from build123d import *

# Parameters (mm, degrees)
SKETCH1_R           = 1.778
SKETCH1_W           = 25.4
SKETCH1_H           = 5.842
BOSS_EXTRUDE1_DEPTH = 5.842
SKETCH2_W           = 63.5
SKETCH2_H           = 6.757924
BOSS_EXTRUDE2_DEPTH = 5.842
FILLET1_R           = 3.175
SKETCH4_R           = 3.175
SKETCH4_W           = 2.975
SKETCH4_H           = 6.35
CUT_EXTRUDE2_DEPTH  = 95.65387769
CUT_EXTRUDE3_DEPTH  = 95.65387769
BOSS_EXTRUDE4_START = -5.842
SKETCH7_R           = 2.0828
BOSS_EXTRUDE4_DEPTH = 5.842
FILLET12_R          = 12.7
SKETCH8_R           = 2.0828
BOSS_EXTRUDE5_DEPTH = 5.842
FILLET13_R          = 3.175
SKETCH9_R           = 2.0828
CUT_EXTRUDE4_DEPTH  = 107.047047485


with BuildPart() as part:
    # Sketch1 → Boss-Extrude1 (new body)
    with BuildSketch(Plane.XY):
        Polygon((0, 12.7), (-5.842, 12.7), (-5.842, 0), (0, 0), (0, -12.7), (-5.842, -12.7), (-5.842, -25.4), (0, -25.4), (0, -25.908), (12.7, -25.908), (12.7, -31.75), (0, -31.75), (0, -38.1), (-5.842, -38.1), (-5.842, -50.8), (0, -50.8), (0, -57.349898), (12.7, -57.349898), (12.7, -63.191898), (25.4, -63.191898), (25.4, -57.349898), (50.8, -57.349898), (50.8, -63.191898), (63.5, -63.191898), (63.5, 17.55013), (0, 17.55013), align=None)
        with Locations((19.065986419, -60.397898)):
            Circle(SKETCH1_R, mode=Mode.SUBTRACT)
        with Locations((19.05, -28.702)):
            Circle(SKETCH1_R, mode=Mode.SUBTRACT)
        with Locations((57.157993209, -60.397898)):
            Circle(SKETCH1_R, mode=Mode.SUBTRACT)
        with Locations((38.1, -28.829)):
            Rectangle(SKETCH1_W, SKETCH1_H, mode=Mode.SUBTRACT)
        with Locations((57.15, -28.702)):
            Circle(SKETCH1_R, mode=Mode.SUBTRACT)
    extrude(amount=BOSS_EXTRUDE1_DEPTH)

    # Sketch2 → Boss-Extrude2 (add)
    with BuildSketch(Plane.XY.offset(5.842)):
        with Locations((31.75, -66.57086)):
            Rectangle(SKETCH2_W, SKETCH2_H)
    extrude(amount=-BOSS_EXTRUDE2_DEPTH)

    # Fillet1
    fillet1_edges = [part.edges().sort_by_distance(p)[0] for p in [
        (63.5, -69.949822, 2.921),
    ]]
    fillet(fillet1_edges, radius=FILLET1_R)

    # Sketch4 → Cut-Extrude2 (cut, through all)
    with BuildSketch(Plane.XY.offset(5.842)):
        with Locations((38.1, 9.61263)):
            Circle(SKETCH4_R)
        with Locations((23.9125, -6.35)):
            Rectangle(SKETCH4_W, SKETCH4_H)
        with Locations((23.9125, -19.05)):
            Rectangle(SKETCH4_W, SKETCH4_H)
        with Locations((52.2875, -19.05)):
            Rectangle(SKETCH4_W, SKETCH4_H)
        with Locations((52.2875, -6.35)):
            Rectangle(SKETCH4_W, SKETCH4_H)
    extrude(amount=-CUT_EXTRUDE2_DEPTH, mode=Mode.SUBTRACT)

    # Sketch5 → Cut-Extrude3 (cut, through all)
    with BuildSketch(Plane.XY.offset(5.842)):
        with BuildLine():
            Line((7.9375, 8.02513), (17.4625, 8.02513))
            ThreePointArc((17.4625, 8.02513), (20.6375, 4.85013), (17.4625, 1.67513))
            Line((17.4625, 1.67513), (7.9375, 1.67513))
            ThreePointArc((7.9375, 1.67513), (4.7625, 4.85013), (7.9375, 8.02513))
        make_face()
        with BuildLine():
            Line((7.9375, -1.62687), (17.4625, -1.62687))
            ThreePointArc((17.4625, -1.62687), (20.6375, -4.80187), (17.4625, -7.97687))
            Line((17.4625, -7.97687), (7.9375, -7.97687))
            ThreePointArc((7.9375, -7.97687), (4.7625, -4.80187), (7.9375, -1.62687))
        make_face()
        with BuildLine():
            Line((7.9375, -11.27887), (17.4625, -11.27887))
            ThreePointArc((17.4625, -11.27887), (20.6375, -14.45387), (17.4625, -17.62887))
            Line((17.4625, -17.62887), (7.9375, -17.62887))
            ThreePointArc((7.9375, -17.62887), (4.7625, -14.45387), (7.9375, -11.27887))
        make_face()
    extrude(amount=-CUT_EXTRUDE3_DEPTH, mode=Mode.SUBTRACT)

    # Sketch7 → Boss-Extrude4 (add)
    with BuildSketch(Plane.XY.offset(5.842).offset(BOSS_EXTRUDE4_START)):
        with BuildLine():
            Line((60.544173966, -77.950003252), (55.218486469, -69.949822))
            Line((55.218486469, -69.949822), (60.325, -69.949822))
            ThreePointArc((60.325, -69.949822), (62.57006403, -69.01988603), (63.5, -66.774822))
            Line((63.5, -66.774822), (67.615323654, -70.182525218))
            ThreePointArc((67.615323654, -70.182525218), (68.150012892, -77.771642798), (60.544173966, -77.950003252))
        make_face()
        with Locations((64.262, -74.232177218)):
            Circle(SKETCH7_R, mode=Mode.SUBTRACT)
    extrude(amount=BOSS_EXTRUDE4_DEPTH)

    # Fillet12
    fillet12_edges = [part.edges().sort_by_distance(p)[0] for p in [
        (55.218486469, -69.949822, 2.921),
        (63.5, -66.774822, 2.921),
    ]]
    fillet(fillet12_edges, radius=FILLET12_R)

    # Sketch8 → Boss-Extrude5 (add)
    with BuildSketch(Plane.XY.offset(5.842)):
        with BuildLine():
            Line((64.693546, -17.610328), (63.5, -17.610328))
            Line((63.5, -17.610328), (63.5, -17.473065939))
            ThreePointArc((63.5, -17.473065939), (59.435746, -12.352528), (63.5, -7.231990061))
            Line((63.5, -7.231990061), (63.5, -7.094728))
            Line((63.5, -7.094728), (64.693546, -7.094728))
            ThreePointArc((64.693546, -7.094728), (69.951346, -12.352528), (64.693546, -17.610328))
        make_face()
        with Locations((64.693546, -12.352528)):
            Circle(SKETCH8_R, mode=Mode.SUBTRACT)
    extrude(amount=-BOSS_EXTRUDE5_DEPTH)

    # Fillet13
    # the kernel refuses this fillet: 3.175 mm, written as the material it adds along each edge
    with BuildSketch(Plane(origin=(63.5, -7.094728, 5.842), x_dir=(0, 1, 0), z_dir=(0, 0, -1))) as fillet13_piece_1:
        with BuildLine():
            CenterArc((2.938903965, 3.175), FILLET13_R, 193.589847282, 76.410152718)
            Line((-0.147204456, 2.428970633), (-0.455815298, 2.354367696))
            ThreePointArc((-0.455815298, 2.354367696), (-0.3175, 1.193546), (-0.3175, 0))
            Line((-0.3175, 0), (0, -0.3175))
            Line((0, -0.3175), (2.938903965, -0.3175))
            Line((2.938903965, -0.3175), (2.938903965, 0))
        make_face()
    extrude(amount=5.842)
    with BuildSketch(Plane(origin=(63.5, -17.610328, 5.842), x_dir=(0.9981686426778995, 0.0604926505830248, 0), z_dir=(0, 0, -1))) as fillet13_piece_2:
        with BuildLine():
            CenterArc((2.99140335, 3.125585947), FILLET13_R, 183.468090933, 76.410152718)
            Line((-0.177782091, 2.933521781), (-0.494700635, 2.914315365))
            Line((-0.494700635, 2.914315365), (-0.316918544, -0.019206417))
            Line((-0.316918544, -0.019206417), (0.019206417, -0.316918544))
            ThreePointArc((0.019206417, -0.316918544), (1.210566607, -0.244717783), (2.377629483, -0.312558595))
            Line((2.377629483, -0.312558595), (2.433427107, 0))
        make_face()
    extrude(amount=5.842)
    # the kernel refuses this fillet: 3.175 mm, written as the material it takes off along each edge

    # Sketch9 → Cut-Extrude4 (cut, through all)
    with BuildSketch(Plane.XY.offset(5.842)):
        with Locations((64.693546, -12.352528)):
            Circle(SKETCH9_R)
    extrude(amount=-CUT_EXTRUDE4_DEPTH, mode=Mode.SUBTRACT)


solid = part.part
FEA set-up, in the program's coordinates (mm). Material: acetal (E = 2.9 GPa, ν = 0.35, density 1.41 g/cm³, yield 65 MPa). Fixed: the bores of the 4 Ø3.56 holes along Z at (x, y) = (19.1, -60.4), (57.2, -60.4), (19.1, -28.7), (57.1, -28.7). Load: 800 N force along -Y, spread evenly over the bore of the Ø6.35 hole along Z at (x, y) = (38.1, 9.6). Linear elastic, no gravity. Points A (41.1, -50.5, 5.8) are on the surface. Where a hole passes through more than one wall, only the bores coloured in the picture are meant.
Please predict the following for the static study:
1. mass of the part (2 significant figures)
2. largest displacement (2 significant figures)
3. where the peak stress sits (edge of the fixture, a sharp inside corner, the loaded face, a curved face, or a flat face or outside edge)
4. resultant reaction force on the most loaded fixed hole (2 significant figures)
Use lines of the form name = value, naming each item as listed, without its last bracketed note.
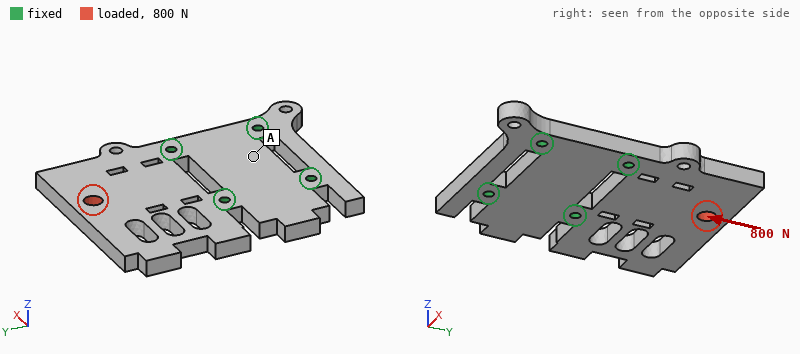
mass of the part = 42 g
largest displacement = 0.12 mm
where the peak stress sits = a curved face
resultant reaction force on the most loaded fixed hole = 390 N
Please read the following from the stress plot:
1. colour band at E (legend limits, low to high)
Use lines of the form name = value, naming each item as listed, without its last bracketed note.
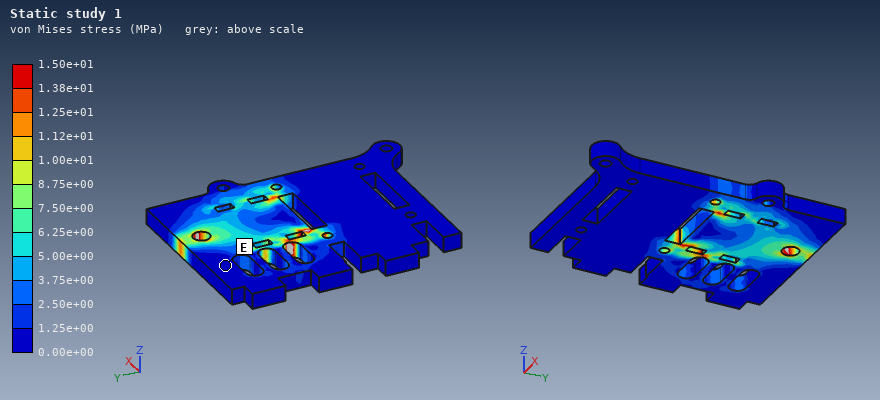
colour band at E = 0.00e+00 to 1.25e+00 MPa
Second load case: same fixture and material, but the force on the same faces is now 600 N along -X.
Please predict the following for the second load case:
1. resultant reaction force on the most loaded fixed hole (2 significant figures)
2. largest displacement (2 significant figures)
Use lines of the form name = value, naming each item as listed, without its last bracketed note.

resultant reaction force on the most loaded fixed hole = 600 N
largest displacement = 0.29 mm
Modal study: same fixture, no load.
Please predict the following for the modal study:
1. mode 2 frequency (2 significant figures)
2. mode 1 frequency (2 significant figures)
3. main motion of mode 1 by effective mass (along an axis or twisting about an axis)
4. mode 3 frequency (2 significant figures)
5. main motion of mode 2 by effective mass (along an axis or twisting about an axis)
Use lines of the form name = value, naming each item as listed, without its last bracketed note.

mode 2 frequency = 860 Hz
mode 1 frequency = 430 Hz
main motion of mode 1 by effective mass = along Z
mode 3 frequency = 1900 Hz
main motion of mode 2 by effective mass = twisting about Y
